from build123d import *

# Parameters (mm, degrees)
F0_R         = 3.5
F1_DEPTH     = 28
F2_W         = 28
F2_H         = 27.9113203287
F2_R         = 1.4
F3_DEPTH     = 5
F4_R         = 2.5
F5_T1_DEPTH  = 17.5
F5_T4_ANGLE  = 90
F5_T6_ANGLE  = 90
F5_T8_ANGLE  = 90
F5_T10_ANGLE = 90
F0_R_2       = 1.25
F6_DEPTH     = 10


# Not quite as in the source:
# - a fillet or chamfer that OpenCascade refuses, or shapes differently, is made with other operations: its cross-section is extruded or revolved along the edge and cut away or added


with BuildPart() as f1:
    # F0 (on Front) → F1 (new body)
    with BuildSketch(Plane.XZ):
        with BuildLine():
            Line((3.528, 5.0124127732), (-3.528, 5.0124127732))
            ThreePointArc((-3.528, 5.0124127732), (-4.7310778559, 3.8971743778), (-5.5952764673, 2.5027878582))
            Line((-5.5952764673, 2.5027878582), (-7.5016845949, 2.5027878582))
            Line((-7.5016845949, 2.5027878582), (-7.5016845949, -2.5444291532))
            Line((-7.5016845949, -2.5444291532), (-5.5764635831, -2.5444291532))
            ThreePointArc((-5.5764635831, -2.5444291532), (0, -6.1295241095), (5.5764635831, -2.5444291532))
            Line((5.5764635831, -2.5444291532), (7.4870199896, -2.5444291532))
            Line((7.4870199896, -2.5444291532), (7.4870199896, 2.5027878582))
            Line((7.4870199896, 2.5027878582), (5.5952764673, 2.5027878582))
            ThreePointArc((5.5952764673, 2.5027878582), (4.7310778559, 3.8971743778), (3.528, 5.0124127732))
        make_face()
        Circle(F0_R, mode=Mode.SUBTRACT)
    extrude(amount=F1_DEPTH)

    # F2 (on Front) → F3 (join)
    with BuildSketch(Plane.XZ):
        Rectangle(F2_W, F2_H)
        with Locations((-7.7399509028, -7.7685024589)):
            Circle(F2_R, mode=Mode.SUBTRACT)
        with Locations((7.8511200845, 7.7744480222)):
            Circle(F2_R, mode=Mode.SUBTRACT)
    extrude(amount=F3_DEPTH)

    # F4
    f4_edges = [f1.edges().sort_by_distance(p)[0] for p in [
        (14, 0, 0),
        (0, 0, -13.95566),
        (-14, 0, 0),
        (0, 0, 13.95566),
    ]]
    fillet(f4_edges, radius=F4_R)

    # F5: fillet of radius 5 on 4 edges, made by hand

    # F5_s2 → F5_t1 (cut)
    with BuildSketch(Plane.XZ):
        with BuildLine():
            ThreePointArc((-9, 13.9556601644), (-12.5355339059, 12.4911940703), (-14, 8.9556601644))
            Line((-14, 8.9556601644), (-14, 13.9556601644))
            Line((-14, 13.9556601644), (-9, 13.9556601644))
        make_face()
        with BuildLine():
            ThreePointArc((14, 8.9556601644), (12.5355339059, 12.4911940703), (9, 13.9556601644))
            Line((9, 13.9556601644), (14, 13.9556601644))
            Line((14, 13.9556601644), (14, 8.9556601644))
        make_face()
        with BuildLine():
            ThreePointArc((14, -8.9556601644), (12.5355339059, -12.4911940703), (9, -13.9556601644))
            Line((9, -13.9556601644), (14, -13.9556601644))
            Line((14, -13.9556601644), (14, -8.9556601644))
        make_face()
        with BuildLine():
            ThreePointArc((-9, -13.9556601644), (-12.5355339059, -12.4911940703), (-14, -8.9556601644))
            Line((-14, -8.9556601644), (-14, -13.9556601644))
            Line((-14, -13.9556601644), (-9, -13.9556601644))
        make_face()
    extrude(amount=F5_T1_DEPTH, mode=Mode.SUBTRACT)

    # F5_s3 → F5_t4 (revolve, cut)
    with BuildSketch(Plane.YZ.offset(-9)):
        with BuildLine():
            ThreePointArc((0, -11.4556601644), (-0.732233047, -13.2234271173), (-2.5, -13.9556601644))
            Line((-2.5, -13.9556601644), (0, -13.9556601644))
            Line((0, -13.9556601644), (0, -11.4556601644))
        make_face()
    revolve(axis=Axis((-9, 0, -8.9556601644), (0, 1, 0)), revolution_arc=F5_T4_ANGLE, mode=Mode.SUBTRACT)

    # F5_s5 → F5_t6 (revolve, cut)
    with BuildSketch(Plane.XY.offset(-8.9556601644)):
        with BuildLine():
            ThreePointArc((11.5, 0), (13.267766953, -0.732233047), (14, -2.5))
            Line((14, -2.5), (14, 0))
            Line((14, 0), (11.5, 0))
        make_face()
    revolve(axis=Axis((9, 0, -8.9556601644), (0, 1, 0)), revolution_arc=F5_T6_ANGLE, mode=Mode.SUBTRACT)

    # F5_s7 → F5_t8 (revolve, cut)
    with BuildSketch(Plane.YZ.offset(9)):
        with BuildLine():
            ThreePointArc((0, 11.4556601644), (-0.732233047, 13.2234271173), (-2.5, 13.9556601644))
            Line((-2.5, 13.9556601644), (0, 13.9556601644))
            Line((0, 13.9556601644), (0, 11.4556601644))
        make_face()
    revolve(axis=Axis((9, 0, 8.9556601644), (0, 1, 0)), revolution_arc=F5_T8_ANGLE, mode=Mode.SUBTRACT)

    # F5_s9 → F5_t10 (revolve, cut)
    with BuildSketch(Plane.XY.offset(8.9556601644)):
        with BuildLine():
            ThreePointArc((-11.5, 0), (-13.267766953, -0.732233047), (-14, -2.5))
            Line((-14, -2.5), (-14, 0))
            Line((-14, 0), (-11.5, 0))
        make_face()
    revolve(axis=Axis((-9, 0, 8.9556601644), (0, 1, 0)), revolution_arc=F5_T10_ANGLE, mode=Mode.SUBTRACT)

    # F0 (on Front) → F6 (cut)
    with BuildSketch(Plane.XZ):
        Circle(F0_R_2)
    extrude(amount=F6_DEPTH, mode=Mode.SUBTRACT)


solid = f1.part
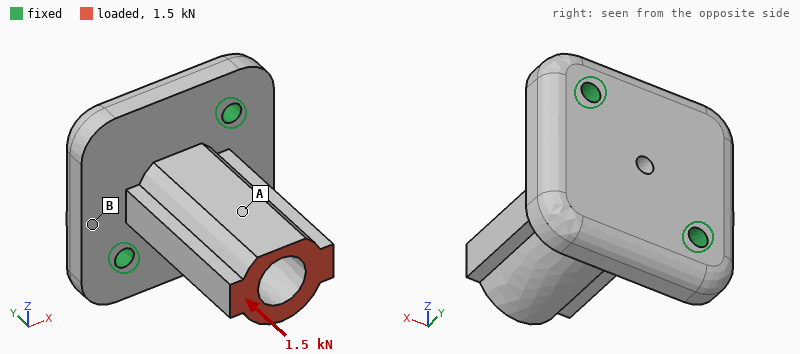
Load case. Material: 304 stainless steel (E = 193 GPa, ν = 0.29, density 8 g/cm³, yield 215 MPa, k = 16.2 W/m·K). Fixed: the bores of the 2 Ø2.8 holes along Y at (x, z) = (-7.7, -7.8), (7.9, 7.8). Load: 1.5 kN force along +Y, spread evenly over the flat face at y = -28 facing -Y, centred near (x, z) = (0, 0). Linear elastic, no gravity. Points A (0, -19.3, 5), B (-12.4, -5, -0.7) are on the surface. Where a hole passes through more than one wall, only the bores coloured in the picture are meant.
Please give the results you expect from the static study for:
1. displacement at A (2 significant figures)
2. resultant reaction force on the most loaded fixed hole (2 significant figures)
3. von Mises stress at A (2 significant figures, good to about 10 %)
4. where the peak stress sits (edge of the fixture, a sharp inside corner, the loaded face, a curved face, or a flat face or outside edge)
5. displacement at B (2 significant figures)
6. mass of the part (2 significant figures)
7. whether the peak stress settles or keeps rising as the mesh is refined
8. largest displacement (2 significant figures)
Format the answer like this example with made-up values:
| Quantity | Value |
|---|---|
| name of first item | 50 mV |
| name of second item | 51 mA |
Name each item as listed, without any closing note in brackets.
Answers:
| Quantity | Value |
|---|---|
| displacement at A | 3.5 µm |
| resultant reaction force on the most loaded fixed hole | 780 N |
| von Mises stress at A | 17 MPa |
| where the peak stress sits | edge of the fixture |
| displacement at B | 1.6 µm |
| mass of the part | 45 g |
| whether the peak stress settles or keeps rising as the mesh is refined | keeps rising |
| largest displacement | 4.5 µm |
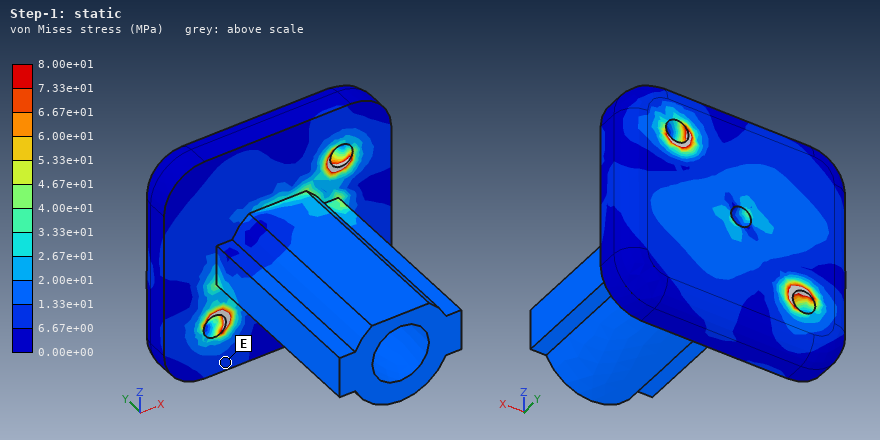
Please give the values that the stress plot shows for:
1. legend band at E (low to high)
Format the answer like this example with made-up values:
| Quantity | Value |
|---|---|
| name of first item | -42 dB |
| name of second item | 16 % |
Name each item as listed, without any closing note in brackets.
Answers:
| Quantity | Value |
|---|---|
| legend band at E | 6.67e+00 to 1.33e+01 MPa |
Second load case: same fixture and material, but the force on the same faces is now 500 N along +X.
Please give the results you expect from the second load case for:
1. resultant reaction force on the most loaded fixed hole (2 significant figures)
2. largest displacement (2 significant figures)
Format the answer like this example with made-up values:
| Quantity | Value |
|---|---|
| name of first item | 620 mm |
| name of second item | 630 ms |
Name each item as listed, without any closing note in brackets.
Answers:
| Quantity | Value |
|---|---|
| resultant reaction force on the most loaded fixed hole | 540 N |
| largest displacement | 28 µm |
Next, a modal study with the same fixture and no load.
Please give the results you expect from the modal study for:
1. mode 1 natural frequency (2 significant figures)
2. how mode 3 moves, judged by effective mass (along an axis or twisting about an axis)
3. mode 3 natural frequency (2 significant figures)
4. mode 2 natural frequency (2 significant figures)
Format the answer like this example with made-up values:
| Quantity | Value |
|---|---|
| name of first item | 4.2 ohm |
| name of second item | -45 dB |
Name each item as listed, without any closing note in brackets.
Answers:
| Quantity | Value |
|---|---|
| mode 1 natural frequency | 6800 Hz |
| how mode 3 moves, judged by effective mass | along Y |
| mode 3 natural frequency | 18 kHz |
| mode 2 natural frequency | 11 kHz |
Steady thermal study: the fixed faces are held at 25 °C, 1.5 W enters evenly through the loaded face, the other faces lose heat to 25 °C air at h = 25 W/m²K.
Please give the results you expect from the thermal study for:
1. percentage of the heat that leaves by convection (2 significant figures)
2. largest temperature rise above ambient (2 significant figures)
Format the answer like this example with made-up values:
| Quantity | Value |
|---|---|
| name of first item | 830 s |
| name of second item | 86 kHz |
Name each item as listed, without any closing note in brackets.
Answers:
| Quantity | Value |
|---|---|
| percentage of the heat that leaves by convection | 37 % |
| largest temperature rise above ambient | 23 K |
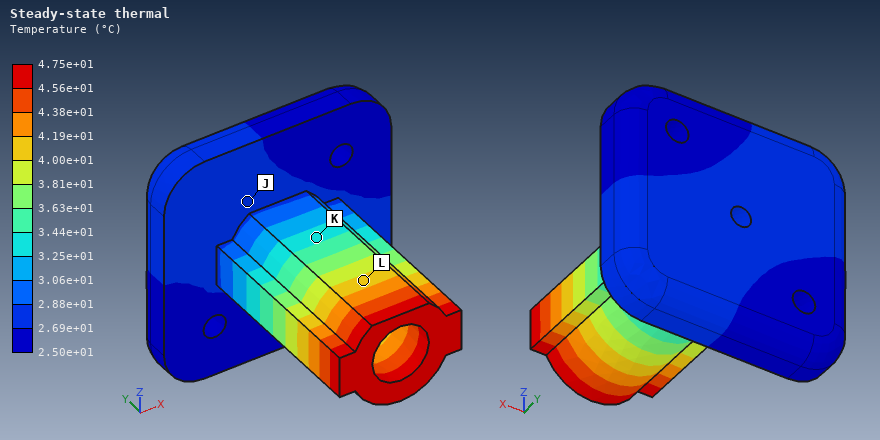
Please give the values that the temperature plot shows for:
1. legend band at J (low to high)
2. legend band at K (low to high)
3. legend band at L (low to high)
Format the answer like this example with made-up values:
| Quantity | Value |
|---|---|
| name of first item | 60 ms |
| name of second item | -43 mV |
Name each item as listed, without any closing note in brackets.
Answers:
| Quantity | Value |
|---|---|
| legend band at J | 2.69e+01 to 2.88e+01 °C |
| legend band at K | 3.25e+01 to 3.44e+01 °C |
| legend band at L | 4.00e+01 to 4.19e+01 °C |
